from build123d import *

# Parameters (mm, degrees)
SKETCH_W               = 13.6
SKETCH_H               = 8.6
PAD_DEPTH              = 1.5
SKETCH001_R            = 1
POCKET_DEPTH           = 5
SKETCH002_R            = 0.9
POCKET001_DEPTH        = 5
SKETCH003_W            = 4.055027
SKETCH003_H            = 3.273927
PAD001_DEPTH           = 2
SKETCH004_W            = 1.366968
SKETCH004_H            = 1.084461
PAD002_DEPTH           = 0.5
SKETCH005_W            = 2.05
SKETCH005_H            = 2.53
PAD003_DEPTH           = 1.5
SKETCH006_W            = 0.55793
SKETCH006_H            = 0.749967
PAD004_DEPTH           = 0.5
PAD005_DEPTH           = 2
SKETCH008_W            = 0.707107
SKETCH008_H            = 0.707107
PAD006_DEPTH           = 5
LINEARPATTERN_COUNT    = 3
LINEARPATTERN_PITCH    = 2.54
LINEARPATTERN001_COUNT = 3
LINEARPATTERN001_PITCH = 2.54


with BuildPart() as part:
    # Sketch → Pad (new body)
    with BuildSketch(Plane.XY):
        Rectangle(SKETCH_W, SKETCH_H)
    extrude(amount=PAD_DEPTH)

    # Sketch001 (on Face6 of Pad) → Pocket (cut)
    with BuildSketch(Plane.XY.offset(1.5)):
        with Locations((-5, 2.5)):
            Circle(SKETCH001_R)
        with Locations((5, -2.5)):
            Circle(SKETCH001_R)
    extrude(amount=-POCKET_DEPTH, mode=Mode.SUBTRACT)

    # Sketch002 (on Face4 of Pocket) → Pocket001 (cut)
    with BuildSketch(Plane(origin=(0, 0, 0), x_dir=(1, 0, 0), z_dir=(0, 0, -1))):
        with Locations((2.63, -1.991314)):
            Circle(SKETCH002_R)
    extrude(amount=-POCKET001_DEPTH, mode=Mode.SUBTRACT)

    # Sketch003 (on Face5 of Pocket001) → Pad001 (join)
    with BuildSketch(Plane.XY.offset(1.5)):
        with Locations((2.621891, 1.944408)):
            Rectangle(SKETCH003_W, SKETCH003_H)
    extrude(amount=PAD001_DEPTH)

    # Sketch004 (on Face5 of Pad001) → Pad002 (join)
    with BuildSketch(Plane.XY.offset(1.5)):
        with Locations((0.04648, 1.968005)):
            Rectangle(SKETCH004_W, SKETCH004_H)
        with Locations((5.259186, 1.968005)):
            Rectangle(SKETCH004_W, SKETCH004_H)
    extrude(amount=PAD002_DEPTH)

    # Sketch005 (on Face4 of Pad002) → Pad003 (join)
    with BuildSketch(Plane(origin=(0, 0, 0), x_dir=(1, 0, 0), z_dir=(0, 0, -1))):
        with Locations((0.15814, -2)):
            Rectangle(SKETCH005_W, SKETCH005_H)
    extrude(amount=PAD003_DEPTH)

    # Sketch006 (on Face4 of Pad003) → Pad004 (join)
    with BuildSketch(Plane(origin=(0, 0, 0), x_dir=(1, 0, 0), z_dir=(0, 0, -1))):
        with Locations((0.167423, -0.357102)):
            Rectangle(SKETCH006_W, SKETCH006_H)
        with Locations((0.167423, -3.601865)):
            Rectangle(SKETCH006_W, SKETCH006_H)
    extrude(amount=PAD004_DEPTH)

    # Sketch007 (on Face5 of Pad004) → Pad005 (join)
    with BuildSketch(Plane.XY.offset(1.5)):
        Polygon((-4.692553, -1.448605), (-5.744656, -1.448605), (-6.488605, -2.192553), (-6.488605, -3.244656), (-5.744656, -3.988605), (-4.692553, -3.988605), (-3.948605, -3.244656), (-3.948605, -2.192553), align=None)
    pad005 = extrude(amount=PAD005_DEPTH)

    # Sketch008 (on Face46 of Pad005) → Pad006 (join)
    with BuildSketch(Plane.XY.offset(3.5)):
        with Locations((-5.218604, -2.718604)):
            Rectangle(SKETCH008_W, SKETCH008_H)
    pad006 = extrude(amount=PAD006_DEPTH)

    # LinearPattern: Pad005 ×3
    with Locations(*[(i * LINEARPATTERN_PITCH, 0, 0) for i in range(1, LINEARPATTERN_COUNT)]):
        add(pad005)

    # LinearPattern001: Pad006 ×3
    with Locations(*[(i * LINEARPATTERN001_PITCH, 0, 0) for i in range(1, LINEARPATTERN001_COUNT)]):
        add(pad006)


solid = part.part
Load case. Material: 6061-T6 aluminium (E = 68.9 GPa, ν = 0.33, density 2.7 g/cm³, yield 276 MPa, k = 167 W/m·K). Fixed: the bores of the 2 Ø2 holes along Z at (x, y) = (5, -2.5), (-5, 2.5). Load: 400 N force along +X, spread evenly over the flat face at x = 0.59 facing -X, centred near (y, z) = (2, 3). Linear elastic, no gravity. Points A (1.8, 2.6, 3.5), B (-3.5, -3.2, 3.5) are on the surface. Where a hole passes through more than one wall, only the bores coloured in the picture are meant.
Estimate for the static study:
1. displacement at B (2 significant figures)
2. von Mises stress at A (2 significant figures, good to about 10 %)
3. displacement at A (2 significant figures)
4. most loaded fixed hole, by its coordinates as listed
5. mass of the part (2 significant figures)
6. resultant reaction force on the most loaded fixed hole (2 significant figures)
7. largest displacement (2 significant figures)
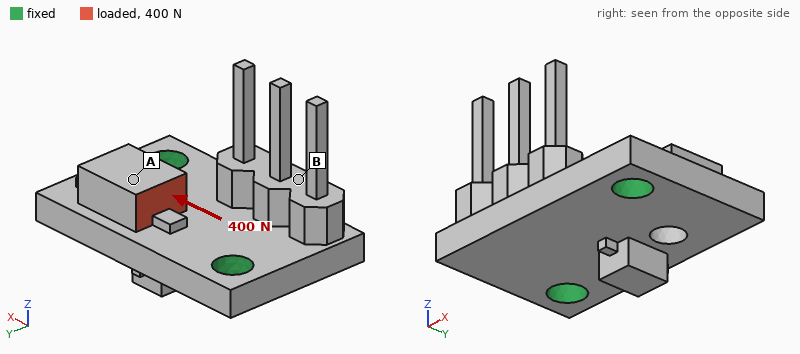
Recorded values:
4.9 µm
61 MPa
15 µm
(-5, 2.5)
0.64 g
240 N
24 µm
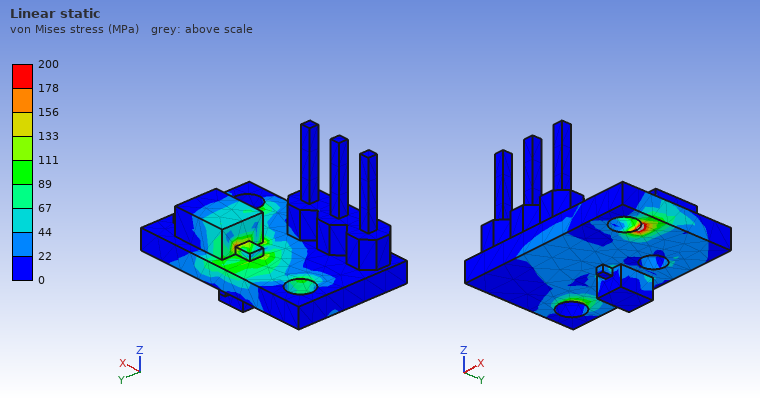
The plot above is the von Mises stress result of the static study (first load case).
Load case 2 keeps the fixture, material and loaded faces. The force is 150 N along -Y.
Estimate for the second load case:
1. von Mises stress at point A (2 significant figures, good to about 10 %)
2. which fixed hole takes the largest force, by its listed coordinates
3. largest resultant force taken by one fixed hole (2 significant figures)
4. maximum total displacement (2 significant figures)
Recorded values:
16 MPa
(5, -2.5)
91 N
17 µm
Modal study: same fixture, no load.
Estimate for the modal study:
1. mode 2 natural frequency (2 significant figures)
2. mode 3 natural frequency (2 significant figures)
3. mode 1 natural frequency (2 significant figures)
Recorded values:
21 kHz
22 kHz
19 kHz
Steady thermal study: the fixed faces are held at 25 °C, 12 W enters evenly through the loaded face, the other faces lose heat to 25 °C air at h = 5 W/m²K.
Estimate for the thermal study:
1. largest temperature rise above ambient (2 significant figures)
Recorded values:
39 K
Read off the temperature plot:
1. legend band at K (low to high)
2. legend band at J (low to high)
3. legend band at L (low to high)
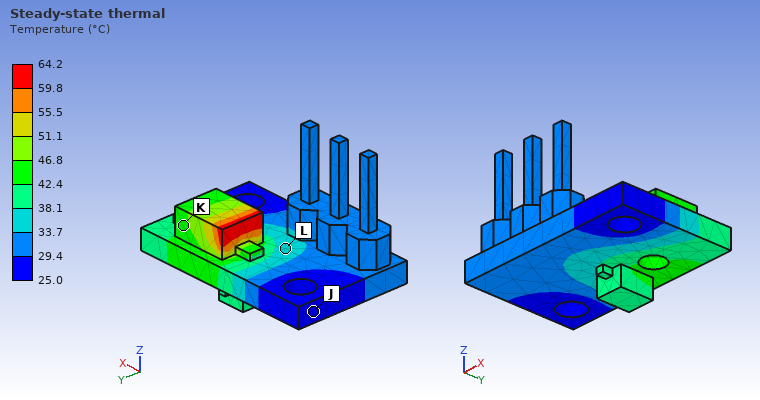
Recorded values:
42.4 to 46.8 °C
25.0 to 29.4 °C
33.7 to 38.1 °C
